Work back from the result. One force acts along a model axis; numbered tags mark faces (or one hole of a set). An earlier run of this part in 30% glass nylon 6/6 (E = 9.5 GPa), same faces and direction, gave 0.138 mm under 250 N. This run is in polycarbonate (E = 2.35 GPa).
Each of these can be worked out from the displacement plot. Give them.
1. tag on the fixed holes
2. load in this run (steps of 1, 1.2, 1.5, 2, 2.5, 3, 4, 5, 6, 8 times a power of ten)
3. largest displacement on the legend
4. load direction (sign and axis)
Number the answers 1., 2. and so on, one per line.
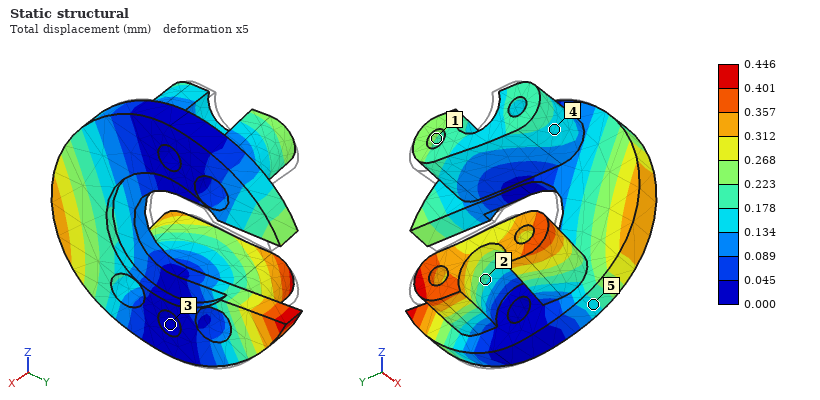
1. 3
2. 200 N
3. 0.446 mm
4. -Y
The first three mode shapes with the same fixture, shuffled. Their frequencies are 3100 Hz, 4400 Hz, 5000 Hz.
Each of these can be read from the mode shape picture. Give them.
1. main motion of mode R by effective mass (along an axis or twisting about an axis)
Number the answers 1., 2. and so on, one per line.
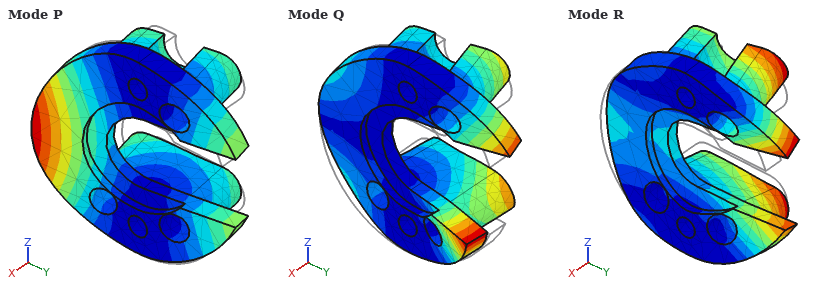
1. along X
